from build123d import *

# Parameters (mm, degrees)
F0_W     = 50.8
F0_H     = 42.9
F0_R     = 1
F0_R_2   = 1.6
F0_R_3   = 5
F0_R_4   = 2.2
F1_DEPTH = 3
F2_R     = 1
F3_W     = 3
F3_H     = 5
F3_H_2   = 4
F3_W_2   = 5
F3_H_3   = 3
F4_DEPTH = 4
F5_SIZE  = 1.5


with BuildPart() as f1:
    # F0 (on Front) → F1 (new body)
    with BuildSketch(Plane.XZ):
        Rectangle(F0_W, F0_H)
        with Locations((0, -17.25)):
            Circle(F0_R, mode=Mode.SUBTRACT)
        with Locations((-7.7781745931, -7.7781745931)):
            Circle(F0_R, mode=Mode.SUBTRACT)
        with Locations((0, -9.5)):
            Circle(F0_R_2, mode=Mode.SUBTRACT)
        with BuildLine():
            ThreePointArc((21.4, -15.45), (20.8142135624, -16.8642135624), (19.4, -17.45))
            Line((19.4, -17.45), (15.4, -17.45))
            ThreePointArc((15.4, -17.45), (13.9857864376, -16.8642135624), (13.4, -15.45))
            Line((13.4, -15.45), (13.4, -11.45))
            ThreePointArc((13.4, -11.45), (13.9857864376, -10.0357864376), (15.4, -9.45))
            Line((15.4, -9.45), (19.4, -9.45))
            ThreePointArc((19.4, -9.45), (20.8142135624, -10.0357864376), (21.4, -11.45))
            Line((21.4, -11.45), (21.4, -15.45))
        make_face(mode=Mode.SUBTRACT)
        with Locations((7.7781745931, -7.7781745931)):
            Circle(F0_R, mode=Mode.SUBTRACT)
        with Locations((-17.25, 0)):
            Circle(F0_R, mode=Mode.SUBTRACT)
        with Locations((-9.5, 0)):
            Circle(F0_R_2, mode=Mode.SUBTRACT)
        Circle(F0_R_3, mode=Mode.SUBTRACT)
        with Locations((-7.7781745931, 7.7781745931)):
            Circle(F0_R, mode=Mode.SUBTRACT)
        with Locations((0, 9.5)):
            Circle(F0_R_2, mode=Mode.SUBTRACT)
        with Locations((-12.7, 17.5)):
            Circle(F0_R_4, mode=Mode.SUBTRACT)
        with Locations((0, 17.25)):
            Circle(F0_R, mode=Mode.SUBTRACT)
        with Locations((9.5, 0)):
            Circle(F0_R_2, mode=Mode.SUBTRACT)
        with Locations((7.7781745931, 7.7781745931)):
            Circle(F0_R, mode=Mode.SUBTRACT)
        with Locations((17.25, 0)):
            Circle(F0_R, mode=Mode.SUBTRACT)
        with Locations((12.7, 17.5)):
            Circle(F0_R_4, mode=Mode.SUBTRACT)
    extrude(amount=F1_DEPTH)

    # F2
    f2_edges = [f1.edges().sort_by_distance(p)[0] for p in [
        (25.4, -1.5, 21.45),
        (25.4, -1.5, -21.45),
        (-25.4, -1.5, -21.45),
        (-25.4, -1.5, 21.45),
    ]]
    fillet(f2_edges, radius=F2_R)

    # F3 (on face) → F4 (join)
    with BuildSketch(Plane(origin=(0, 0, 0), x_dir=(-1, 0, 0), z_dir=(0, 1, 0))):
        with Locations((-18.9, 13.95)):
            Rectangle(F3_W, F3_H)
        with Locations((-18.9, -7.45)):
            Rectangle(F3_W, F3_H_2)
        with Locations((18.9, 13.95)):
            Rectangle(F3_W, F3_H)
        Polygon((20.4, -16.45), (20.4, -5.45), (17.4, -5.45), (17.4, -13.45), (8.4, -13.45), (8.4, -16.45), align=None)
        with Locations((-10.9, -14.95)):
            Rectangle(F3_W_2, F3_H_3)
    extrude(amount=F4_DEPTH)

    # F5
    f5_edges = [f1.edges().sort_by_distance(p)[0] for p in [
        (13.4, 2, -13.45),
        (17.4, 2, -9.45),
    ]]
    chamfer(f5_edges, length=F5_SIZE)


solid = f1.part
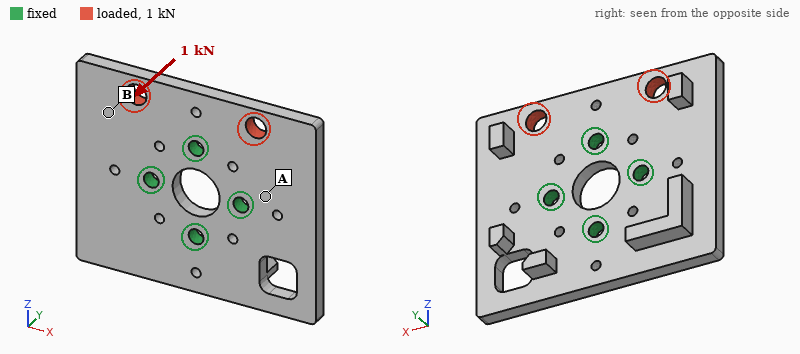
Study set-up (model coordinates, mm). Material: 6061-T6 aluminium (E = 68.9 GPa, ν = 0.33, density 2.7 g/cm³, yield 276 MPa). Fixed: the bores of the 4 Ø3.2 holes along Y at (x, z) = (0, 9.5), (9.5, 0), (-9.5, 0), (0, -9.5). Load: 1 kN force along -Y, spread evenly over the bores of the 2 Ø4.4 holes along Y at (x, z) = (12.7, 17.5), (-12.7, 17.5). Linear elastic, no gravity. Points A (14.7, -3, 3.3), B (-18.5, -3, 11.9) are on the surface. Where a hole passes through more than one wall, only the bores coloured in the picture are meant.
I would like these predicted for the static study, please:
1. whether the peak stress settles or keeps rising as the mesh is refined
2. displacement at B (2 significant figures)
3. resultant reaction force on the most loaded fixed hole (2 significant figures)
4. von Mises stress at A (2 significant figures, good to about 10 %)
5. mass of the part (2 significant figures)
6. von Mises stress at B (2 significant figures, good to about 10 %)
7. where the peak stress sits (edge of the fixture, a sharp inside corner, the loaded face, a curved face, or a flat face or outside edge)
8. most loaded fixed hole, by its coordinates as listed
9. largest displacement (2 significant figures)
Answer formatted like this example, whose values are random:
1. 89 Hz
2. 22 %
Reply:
1. keeps rising
2. 0.090 mm
3. 830 N
4. 77 MPa
5. 17 g
6. 37 MPa
7. edge of the fixture
8. (0, 9.5)
9. 0.21 mm
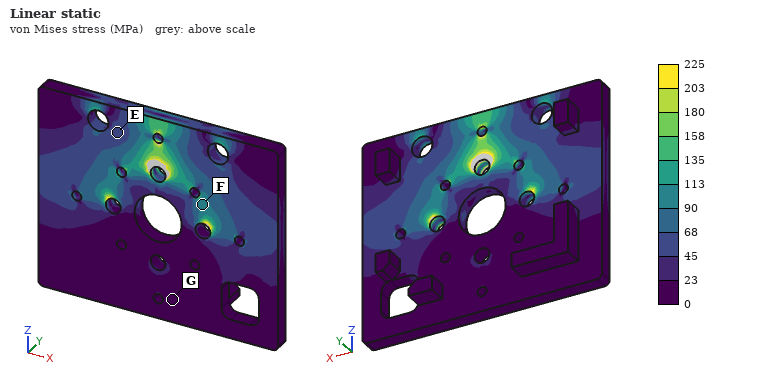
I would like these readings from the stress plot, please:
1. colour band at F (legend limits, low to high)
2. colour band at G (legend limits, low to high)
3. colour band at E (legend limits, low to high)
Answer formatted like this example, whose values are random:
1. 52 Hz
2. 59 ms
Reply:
1. 90 to 113 MPa
2. 0 to 23 MPa
3. 45 to 68 MPa
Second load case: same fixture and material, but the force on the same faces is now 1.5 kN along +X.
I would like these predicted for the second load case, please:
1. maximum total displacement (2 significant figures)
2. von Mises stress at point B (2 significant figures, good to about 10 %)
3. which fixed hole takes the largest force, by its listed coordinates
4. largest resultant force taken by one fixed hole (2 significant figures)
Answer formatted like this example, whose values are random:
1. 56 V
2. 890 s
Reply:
1. 14 µm
2. 9.8 MPa
3. (0, 9.5)
4. 1.4 kN
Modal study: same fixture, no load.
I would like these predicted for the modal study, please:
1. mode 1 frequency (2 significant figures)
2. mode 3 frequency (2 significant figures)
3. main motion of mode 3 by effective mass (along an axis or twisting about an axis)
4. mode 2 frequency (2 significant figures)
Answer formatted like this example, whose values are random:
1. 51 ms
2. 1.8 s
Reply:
1. 5500 Hz
2. 6100 Hz
3. along Y
4. 5700 Hz
